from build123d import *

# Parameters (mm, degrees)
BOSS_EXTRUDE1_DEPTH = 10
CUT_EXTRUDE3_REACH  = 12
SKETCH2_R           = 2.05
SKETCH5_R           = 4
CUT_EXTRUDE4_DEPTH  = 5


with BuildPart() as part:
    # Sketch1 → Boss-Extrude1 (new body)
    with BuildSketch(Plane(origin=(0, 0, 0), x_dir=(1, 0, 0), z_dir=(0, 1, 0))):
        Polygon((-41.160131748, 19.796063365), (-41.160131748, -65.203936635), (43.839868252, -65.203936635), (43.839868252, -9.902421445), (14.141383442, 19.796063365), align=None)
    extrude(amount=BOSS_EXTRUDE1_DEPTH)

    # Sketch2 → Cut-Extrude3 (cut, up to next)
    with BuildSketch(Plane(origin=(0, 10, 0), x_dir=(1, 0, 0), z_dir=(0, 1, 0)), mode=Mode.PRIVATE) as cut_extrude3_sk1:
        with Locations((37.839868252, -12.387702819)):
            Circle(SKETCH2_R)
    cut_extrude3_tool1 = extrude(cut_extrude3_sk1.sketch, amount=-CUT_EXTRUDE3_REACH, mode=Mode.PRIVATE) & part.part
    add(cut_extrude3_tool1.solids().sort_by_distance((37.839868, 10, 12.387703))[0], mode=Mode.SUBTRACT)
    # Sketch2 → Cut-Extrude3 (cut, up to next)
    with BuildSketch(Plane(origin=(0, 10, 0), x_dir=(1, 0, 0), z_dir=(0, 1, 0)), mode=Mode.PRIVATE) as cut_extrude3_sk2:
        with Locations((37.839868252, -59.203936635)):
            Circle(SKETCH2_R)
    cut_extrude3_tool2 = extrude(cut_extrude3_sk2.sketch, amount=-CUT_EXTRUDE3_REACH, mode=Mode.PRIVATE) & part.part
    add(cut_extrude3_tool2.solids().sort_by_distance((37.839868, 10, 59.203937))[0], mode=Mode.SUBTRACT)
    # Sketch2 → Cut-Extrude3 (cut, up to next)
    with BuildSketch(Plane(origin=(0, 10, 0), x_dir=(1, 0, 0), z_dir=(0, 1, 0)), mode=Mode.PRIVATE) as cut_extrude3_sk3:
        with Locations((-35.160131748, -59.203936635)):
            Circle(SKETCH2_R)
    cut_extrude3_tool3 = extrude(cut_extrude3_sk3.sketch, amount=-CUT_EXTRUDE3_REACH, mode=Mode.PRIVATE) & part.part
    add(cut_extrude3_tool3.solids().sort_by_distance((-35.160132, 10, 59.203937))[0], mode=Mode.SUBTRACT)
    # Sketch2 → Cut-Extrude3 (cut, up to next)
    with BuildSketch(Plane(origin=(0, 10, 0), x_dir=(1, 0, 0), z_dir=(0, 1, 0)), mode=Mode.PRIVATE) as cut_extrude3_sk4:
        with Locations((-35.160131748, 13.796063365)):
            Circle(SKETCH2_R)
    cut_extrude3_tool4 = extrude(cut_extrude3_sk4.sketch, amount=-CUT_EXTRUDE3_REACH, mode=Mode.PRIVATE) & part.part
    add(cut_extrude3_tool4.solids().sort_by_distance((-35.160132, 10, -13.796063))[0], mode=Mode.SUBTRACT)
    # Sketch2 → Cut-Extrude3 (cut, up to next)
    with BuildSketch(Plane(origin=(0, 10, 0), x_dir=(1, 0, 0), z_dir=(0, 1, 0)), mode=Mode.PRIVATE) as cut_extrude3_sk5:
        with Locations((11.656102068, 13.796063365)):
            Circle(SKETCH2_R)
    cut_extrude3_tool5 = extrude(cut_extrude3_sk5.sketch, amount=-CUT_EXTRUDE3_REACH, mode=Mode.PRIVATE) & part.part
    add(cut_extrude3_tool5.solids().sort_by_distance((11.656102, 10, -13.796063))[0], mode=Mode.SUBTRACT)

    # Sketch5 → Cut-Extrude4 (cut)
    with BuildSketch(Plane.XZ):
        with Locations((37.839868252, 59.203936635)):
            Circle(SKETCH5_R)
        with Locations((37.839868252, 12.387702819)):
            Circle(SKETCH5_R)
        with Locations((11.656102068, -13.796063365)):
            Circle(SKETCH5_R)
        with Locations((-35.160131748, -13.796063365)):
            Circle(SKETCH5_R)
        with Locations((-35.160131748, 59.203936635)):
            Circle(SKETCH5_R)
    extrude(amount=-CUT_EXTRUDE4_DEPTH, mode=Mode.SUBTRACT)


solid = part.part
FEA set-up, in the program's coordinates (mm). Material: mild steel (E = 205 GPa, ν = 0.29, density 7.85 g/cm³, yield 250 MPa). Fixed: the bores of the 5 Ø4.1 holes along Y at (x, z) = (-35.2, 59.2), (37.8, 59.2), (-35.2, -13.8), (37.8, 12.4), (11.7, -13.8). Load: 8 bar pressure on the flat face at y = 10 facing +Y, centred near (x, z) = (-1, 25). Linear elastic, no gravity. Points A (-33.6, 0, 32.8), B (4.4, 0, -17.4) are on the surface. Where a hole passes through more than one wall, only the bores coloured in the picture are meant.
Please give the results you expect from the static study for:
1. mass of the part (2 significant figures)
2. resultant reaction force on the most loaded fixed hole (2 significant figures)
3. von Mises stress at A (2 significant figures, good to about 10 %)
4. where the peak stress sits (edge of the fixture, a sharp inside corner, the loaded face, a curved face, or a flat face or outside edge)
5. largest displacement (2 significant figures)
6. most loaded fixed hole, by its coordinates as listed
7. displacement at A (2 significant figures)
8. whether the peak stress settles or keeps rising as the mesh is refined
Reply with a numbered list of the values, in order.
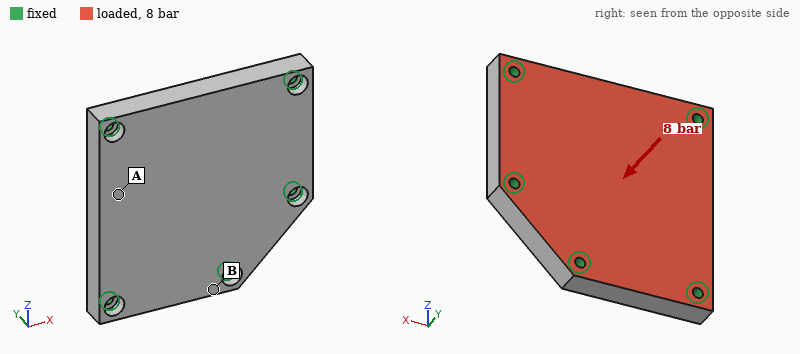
1. 520 g
2. 1.9 kN
3. 20 MPa
4. edge of the fixture
5. 12 µm
6. (-35.2, 59.2)
7. 8.9 µm
8. keeps rising
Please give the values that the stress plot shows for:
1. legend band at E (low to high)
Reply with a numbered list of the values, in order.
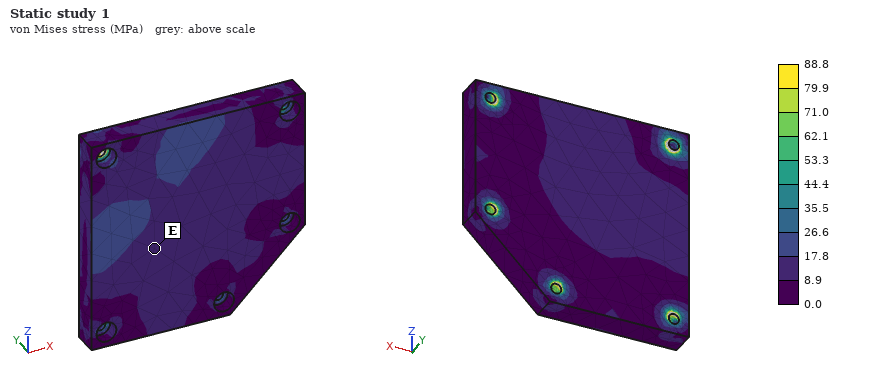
1. 8.9 to 17.8 MPa
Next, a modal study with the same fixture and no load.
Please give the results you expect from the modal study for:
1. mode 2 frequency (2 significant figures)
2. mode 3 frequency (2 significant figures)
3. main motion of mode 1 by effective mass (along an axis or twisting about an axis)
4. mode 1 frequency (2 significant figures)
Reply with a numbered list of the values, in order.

1. 8100 Hz
2. 12 kHz
3. along Y
4. 5500 Hz
